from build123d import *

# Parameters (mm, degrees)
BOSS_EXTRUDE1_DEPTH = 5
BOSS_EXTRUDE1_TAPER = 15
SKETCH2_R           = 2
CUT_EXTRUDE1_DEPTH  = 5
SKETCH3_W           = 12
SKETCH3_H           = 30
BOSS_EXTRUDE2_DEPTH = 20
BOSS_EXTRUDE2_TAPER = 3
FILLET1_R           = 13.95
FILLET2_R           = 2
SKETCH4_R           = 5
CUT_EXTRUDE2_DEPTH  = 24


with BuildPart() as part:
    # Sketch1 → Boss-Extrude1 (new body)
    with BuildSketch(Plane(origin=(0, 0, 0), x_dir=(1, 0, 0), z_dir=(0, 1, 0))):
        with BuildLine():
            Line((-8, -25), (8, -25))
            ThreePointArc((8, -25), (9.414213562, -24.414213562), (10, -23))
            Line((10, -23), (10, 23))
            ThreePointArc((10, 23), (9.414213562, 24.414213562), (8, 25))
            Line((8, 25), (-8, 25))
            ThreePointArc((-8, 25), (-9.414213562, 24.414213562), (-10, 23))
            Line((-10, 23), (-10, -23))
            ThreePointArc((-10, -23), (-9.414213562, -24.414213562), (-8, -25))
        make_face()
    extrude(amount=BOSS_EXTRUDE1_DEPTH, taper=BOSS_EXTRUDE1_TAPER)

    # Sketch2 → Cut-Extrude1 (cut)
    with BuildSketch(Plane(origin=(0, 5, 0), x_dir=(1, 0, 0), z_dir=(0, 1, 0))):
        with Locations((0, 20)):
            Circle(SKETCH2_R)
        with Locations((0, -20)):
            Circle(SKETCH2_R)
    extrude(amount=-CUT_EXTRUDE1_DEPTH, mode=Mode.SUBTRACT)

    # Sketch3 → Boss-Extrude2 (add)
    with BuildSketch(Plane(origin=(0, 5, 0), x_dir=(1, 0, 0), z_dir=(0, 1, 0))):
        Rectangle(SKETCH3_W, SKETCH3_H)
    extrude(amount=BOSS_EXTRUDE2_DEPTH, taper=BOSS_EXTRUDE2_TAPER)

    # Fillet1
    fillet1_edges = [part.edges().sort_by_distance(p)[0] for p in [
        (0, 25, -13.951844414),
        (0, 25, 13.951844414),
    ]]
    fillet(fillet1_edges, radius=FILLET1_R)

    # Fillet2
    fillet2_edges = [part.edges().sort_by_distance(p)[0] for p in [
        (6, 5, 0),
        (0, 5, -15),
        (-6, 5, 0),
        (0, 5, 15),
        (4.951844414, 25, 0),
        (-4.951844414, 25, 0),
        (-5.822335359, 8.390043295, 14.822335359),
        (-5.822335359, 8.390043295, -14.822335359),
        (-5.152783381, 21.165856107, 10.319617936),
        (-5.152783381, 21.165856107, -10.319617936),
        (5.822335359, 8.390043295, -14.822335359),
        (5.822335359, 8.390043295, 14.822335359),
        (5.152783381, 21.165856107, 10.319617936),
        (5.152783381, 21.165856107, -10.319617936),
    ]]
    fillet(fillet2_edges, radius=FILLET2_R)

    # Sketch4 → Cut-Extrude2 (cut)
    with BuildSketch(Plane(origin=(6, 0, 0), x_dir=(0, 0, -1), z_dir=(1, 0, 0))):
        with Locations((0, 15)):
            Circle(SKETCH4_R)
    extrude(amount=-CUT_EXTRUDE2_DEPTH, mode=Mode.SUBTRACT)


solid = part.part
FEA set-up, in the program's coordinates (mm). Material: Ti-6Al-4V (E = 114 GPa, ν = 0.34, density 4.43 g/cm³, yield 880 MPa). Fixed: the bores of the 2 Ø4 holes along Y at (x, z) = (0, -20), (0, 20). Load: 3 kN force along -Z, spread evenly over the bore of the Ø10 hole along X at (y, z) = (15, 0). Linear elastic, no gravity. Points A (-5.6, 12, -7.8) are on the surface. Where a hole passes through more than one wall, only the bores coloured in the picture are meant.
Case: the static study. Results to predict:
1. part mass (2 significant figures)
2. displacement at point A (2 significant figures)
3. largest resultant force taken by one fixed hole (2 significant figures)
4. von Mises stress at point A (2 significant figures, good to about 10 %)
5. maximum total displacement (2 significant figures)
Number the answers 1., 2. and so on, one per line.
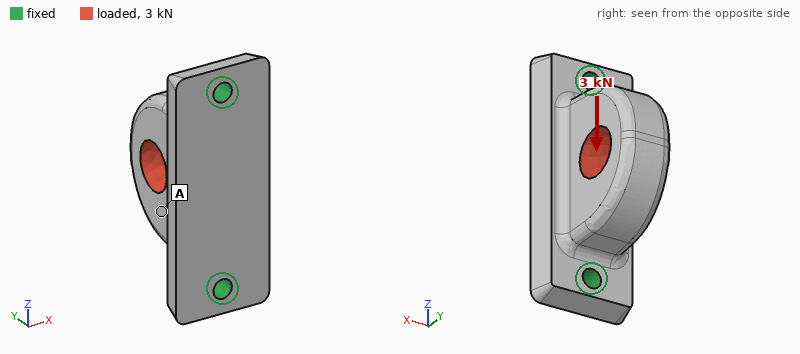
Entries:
1. 40 g
2. 5.3 µm
3. 1.8 kN
4. 19 MPa
5. 11 µm
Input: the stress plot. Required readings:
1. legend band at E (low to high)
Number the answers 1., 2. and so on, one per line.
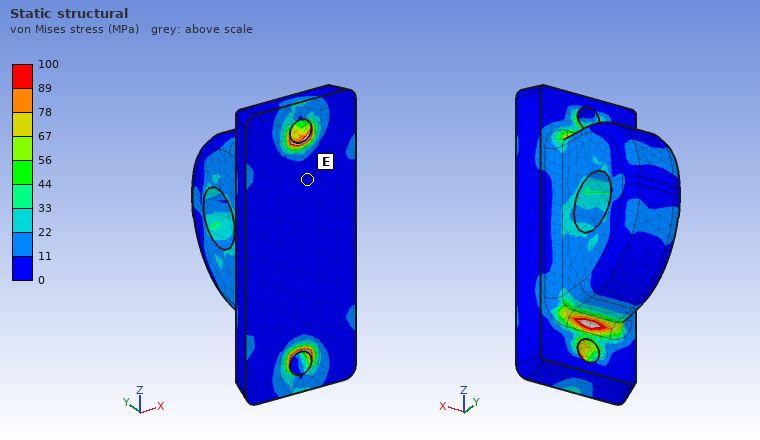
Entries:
1. 0 to 11 MPa
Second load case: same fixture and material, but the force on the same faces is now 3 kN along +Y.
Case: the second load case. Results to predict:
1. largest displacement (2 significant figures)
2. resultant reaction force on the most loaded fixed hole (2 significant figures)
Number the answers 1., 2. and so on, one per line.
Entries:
1. 10.0 µm
2. 1.7 kN
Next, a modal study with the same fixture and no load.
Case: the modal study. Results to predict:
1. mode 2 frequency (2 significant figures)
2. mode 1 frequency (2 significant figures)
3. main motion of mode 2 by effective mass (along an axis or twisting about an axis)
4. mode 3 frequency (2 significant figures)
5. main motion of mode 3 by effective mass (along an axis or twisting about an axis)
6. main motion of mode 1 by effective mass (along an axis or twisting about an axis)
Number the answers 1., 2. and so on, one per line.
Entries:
1. 17 kHz
2. 7400 Hz
3. along Y
4. 22 kHz
5. along Z
6. along X
